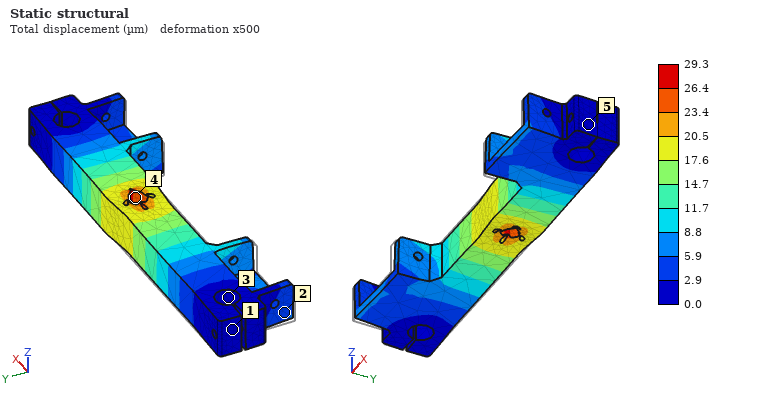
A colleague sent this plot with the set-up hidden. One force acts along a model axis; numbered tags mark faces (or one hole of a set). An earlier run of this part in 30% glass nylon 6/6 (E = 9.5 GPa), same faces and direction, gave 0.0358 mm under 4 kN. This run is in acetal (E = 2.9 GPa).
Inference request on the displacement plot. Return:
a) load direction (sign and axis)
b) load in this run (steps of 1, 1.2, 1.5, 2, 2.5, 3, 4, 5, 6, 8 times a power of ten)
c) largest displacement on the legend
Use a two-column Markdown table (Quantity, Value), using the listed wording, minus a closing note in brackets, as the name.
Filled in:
| Quantity | Value |
|---|---|
| load direction | +X |
| load in this run | 1 kN |
| largest displacement on the legend | 29.3 µm |
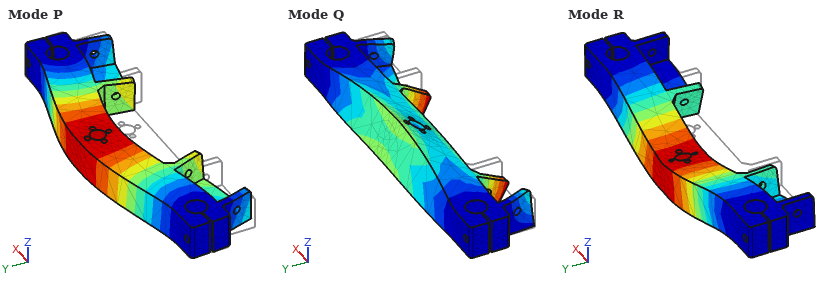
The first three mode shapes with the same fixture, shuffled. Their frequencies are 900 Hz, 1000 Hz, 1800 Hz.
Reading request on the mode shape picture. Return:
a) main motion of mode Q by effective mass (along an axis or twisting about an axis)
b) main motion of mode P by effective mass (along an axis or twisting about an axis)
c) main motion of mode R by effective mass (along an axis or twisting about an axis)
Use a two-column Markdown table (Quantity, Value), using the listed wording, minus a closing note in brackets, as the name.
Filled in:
| Quantity | Value |
|---|---|
| main motion of mode Q by effective mass | twisting about X |
| main motion of mode P by effective mass | along Y |
| main motion of mode R by effective mass | along Z |
